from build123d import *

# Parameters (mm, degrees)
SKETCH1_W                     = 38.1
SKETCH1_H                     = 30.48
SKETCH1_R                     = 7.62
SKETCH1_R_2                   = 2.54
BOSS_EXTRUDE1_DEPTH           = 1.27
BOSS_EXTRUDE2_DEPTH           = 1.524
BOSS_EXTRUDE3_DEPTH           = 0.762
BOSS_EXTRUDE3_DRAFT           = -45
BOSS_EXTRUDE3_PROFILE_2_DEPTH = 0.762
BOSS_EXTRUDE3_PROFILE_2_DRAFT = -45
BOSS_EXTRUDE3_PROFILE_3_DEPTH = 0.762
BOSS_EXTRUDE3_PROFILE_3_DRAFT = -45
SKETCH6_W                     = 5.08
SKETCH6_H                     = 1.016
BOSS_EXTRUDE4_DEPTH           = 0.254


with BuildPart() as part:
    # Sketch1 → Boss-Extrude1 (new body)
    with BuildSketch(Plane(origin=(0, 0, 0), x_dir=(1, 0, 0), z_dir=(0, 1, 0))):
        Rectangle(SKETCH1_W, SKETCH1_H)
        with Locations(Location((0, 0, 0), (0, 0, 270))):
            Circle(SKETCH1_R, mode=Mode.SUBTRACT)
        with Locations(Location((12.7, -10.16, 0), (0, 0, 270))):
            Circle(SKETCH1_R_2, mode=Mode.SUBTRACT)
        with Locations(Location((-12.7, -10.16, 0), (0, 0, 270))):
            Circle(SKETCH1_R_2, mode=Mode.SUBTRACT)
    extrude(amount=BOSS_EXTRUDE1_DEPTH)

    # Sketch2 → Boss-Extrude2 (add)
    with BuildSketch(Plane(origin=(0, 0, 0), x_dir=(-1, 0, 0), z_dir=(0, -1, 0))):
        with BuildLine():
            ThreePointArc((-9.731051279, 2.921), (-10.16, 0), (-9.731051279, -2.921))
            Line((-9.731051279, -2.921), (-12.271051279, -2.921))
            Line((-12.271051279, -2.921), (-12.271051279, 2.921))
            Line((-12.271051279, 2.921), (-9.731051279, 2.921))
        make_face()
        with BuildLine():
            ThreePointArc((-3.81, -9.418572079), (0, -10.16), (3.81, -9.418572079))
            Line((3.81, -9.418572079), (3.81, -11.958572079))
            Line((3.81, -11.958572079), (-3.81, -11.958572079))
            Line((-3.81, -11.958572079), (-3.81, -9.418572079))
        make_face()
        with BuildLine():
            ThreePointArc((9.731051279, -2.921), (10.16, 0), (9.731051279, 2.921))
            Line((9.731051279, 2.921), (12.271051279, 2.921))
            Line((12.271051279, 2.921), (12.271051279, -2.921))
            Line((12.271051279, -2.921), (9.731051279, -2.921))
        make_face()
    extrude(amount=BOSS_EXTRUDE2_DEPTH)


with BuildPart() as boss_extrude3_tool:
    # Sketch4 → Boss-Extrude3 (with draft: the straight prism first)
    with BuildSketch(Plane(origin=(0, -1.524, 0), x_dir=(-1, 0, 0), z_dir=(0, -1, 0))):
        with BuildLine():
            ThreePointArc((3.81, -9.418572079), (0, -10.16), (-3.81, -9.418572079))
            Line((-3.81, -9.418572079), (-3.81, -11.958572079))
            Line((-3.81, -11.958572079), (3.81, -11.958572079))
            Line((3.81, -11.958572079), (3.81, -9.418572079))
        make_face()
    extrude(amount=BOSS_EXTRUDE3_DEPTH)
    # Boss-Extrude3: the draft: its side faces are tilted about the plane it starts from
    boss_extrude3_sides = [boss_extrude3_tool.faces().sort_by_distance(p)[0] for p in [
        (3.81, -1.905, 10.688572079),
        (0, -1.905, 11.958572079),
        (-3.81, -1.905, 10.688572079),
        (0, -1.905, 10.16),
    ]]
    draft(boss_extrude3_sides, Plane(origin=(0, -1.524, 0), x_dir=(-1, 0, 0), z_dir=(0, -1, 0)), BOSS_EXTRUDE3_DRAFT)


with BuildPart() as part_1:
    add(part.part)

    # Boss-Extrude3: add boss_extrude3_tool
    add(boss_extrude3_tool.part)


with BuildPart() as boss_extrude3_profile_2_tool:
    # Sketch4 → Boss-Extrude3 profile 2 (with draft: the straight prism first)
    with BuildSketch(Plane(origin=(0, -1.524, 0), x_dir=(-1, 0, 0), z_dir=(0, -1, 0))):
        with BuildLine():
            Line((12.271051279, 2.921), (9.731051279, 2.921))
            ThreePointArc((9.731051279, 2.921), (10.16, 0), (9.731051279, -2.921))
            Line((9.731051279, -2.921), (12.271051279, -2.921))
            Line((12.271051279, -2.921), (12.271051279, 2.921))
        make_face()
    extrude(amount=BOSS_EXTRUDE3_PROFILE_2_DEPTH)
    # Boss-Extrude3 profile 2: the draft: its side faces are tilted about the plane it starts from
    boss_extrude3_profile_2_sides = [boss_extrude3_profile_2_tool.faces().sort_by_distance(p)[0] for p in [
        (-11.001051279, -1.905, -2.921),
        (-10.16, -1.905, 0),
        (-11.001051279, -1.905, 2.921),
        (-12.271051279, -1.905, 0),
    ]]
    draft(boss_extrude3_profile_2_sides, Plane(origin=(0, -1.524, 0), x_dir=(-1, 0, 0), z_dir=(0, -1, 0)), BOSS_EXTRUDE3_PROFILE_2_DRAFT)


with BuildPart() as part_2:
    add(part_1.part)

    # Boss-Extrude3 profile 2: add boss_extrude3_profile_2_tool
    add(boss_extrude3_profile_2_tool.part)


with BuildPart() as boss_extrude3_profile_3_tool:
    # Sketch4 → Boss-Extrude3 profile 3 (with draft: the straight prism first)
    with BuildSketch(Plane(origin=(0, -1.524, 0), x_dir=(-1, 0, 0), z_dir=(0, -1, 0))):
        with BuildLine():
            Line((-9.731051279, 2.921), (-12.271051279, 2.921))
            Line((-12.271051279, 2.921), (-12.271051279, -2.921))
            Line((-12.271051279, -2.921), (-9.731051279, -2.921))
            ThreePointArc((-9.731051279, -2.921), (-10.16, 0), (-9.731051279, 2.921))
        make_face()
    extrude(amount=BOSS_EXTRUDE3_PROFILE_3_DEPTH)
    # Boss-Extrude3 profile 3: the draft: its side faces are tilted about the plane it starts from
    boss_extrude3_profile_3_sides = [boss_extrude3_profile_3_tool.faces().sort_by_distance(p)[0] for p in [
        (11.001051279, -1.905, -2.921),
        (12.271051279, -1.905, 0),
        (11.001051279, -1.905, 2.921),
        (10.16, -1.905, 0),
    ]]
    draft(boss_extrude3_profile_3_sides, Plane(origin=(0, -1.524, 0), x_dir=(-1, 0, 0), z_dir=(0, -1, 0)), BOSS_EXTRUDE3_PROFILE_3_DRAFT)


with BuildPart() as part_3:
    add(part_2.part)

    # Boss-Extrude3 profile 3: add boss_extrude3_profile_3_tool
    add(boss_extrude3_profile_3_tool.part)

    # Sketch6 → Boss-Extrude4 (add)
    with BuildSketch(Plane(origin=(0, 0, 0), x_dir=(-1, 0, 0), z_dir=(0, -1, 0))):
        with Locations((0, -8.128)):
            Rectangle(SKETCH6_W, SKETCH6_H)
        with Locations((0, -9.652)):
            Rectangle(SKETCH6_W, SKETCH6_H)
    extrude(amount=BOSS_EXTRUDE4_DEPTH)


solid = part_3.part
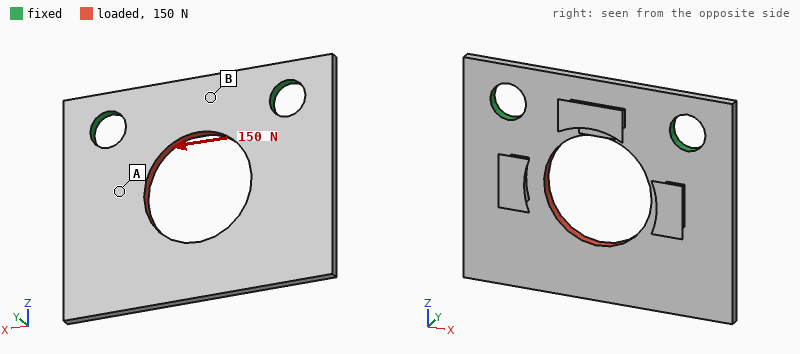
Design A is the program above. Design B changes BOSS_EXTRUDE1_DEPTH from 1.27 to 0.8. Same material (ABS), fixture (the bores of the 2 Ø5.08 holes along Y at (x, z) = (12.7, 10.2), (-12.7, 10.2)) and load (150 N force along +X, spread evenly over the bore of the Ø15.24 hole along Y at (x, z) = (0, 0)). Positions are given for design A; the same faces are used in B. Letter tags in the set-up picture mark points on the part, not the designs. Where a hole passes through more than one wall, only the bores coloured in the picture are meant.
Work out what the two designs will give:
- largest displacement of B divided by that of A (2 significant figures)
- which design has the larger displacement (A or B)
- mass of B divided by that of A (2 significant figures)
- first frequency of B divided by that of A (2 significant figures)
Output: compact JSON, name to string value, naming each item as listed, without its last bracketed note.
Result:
{"largest displacement of B divided by that of A": "1.6", "which design has the larger displacement": "B", "mass of B divided by that of A": "0.66", "first frequency of B divided by that of A": "0.65"}
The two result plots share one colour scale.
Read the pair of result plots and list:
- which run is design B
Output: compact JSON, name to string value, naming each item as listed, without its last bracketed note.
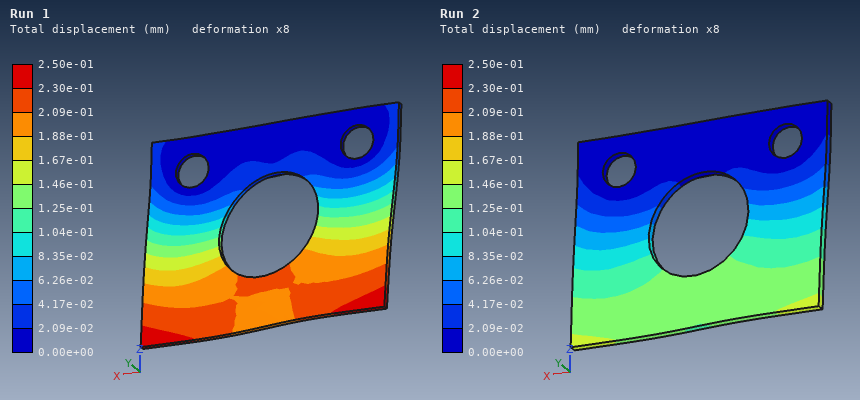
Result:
{"which run is design B": "Run 1"}
